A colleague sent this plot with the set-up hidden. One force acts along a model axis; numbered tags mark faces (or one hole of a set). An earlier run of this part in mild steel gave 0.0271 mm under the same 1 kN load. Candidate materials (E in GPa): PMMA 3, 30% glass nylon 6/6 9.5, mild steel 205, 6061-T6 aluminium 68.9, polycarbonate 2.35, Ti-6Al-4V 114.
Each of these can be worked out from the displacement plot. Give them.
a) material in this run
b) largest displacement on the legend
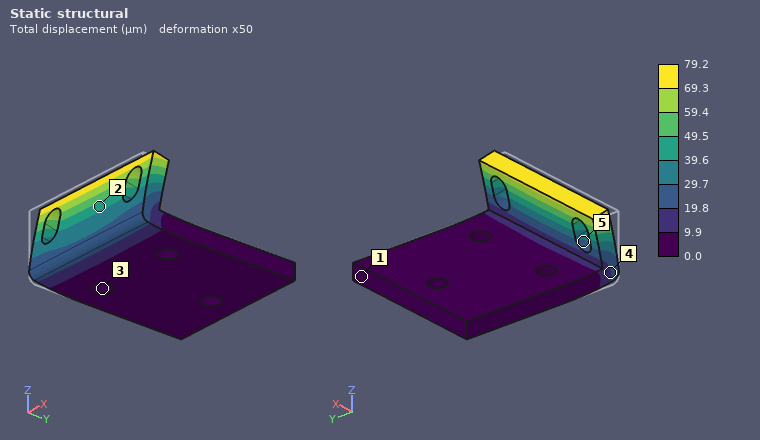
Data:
6061-T6 aluminium
79.2 µm
